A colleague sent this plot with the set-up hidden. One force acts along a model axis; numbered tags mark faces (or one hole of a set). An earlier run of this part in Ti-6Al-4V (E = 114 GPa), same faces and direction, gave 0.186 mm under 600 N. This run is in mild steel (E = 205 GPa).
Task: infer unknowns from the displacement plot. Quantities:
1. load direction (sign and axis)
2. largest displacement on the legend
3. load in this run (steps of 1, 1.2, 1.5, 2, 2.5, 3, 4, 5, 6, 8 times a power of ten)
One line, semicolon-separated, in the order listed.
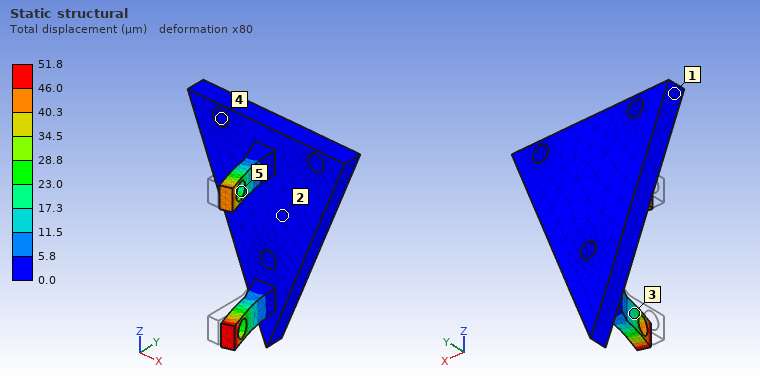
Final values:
+X; 51.8 µm; 300 N
